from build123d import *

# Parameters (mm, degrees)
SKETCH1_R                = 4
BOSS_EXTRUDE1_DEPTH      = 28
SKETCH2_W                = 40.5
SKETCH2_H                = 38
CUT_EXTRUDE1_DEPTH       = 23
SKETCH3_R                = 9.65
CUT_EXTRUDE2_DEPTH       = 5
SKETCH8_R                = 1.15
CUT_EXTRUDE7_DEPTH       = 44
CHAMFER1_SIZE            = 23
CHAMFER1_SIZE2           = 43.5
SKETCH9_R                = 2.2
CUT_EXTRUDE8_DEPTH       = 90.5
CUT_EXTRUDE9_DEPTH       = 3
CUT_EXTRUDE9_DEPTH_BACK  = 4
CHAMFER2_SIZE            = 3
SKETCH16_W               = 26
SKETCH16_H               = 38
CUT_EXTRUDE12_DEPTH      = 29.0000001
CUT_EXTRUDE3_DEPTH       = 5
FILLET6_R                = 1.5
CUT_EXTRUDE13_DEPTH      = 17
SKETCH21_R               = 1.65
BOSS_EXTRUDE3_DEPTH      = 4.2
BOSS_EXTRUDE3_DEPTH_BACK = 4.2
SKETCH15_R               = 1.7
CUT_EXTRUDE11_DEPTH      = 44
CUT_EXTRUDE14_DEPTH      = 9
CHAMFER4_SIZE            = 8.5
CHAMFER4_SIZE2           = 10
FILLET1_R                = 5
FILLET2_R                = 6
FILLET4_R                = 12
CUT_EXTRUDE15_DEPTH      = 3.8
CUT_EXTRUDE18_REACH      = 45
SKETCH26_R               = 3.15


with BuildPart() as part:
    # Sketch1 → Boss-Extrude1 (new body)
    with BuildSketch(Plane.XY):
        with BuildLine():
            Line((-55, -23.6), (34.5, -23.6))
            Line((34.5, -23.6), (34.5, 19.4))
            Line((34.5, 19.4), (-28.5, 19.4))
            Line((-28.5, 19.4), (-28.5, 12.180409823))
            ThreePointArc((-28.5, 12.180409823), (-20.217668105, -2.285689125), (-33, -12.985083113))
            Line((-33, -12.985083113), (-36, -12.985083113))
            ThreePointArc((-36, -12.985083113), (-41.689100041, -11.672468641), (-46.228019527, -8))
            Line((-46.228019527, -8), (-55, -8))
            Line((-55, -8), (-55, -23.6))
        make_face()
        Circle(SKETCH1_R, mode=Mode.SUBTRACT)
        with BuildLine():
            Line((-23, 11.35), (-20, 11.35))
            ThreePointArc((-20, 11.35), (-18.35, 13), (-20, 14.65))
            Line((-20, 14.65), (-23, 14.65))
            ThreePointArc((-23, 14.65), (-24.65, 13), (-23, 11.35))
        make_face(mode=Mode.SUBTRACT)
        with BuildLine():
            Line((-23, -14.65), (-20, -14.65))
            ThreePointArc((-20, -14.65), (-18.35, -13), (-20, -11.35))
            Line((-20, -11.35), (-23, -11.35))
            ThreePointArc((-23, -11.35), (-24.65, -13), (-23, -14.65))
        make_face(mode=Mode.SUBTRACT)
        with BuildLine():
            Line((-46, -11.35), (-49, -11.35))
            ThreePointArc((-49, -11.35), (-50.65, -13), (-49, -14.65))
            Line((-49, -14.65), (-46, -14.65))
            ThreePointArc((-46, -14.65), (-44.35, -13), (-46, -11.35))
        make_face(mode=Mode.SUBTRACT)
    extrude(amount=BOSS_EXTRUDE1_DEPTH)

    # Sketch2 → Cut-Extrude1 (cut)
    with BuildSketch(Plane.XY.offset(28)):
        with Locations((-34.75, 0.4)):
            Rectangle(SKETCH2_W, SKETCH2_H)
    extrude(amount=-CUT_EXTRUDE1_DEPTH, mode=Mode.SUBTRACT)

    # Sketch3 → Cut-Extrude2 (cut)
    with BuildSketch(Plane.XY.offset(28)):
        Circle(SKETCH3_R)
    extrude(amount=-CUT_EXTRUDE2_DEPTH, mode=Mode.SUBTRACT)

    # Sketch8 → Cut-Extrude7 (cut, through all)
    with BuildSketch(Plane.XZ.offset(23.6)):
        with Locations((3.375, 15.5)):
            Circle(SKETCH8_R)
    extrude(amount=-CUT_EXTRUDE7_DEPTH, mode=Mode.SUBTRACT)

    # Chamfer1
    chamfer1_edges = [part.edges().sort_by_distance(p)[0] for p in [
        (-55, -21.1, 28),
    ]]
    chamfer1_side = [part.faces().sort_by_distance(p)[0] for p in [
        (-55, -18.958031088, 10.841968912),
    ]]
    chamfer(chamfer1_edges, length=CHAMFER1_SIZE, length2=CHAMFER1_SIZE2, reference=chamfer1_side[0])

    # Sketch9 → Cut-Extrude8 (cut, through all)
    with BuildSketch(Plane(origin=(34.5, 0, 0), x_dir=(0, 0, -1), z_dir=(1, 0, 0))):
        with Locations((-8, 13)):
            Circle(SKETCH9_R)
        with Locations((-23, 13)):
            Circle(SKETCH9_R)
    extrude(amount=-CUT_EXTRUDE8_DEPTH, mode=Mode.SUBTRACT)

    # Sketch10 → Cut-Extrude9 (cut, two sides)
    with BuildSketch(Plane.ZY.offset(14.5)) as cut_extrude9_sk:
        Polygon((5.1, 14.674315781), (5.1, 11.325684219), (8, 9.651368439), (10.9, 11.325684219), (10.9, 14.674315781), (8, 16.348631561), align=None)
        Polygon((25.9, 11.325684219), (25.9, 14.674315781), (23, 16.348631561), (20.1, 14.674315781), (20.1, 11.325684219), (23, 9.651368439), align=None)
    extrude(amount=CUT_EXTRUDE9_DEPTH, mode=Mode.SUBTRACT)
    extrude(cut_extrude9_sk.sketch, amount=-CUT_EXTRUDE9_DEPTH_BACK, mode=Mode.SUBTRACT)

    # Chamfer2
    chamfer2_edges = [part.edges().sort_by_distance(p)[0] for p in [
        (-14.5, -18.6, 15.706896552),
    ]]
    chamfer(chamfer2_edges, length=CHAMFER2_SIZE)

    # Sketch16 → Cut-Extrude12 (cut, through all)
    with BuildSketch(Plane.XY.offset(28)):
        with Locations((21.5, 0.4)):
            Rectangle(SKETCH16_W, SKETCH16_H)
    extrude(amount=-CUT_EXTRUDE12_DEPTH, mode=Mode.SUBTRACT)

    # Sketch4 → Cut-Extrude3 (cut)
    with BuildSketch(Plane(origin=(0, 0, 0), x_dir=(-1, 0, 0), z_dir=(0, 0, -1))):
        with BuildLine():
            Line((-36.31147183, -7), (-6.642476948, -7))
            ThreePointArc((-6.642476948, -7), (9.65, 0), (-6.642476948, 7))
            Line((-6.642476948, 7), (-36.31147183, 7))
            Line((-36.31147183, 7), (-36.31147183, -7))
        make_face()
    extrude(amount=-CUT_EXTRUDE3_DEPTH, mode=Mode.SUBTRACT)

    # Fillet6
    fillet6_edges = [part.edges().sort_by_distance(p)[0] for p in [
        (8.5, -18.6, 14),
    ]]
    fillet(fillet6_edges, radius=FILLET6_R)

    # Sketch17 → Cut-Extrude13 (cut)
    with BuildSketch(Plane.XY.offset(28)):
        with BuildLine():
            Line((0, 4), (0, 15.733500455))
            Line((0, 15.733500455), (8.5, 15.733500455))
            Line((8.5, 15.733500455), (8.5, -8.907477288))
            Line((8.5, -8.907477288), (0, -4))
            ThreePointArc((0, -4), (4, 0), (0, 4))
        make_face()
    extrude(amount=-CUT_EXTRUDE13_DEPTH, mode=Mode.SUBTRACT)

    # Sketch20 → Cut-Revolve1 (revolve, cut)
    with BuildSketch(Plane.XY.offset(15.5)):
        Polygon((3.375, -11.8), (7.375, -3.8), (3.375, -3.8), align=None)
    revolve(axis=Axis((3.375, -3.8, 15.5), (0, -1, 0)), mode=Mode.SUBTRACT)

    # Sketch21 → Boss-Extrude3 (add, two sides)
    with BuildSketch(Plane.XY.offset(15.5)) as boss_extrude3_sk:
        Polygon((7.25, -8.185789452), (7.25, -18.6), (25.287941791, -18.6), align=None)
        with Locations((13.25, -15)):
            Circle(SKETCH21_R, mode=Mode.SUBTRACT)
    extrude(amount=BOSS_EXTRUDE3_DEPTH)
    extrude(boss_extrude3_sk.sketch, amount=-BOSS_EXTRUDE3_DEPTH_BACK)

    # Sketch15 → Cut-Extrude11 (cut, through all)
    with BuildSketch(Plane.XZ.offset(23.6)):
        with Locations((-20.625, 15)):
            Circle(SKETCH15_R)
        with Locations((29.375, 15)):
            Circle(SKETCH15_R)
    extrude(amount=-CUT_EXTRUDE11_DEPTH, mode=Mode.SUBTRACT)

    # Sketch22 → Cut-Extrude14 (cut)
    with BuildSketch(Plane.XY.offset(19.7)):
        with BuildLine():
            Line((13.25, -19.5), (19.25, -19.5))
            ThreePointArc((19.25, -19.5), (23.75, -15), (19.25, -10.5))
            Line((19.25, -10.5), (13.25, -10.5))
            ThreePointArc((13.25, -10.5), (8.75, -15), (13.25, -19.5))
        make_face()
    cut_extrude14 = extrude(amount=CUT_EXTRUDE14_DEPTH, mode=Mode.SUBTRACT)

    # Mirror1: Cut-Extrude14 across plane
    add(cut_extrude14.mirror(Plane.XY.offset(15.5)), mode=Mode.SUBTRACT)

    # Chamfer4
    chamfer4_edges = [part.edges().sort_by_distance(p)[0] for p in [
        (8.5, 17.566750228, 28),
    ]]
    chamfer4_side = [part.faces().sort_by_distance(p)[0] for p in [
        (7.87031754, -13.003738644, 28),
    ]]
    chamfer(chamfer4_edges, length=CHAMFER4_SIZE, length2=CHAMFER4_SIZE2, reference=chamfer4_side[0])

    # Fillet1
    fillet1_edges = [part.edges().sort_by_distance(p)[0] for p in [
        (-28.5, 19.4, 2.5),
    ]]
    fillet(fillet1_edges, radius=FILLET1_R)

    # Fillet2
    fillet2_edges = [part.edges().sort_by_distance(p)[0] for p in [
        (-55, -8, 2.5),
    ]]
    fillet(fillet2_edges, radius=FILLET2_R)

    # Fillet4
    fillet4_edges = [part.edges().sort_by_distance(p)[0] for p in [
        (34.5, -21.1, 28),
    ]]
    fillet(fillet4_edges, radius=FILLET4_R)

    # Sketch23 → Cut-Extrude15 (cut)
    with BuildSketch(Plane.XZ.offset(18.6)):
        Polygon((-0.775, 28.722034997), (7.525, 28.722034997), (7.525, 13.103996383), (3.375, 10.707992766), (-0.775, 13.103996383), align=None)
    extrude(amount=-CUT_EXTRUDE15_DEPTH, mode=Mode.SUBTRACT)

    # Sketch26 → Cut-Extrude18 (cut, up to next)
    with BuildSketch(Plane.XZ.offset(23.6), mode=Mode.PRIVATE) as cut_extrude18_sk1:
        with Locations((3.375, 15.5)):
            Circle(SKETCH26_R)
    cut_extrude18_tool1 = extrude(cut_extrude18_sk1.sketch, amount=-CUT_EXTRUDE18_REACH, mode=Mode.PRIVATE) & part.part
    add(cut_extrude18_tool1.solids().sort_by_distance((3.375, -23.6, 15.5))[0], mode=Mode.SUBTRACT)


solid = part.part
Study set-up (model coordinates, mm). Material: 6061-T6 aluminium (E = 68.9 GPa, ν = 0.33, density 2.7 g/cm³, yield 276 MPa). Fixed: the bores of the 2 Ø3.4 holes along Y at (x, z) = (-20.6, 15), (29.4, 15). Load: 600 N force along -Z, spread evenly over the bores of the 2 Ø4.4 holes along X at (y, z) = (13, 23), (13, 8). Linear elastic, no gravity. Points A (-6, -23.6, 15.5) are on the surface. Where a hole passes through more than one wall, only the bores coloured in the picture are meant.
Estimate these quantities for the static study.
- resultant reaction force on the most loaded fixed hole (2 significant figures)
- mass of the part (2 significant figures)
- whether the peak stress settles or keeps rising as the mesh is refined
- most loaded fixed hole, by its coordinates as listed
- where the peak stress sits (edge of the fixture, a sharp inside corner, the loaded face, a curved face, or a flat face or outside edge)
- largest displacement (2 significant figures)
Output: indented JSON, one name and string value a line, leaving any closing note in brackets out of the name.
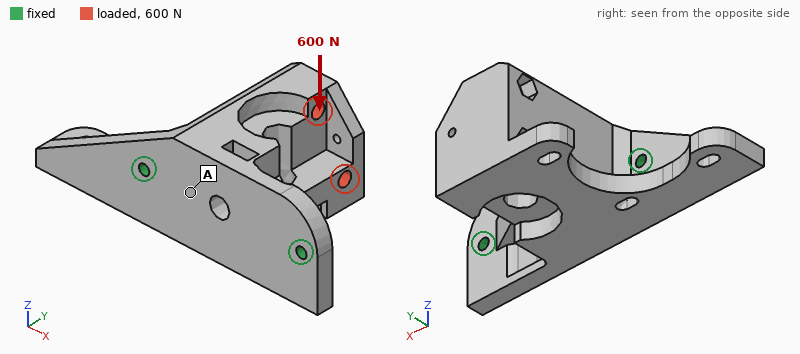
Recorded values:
{
  "resultant reaction force on the most loaded fixed hole": "400 N",
  "mass of the part": "80 g",
  "whether the peak stress settles or keeps rising as the mesh is refined": "keeps rising",
  "most loaded fixed hole, by its coordinates as listed": "(-20.6, 15)",
  "where the peak stress sits": "edge of the fixture",
  "largest displacement": "0.18 mm"
}
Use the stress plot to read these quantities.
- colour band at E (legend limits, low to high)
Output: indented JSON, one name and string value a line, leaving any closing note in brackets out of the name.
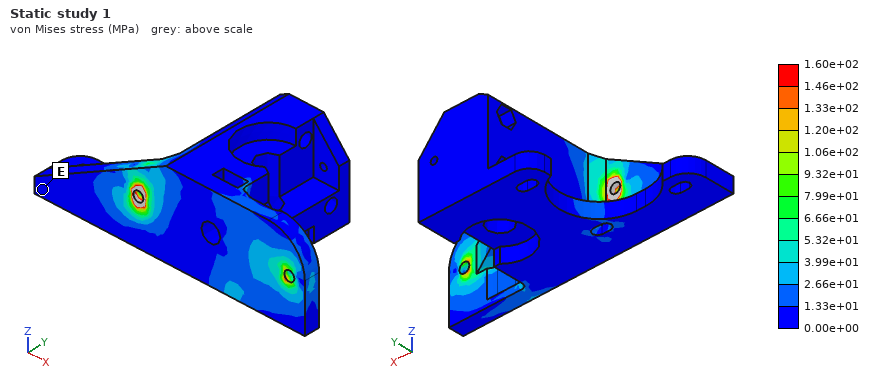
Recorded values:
{
  "colour band at E": "0.00e+00 to 1.33e+01 MPa"
}
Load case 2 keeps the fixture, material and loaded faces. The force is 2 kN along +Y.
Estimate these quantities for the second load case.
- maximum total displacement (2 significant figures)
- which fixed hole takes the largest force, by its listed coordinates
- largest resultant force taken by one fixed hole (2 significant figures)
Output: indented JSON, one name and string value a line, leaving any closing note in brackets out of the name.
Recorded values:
{
  "maximum total displacement": "48 µm",
  "which fixed hole takes the largest force, by its listed coordinates": "(-20.6, 15)",
  "largest resultant force taken by one fixed hole": "1.4 kN"
}
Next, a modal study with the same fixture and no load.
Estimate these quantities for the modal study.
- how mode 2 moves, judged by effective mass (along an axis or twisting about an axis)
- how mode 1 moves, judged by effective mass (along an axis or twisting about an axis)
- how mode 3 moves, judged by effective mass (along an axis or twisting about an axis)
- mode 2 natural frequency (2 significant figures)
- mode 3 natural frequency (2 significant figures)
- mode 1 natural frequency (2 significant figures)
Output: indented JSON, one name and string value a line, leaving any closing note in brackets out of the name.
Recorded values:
{
  "how mode 2 moves, judged by effective mass": "along X",
  "how mode 1 moves, judged by effective mass": "along Z",
  "how mode 3 moves, judged by effective mass": "along Y",
  "mode 2 natural frequency": "4600 Hz",
  "mode 3 natural frequency": "6200 Hz",
  "mode 1 natural frequency": "1900 Hz"
}
